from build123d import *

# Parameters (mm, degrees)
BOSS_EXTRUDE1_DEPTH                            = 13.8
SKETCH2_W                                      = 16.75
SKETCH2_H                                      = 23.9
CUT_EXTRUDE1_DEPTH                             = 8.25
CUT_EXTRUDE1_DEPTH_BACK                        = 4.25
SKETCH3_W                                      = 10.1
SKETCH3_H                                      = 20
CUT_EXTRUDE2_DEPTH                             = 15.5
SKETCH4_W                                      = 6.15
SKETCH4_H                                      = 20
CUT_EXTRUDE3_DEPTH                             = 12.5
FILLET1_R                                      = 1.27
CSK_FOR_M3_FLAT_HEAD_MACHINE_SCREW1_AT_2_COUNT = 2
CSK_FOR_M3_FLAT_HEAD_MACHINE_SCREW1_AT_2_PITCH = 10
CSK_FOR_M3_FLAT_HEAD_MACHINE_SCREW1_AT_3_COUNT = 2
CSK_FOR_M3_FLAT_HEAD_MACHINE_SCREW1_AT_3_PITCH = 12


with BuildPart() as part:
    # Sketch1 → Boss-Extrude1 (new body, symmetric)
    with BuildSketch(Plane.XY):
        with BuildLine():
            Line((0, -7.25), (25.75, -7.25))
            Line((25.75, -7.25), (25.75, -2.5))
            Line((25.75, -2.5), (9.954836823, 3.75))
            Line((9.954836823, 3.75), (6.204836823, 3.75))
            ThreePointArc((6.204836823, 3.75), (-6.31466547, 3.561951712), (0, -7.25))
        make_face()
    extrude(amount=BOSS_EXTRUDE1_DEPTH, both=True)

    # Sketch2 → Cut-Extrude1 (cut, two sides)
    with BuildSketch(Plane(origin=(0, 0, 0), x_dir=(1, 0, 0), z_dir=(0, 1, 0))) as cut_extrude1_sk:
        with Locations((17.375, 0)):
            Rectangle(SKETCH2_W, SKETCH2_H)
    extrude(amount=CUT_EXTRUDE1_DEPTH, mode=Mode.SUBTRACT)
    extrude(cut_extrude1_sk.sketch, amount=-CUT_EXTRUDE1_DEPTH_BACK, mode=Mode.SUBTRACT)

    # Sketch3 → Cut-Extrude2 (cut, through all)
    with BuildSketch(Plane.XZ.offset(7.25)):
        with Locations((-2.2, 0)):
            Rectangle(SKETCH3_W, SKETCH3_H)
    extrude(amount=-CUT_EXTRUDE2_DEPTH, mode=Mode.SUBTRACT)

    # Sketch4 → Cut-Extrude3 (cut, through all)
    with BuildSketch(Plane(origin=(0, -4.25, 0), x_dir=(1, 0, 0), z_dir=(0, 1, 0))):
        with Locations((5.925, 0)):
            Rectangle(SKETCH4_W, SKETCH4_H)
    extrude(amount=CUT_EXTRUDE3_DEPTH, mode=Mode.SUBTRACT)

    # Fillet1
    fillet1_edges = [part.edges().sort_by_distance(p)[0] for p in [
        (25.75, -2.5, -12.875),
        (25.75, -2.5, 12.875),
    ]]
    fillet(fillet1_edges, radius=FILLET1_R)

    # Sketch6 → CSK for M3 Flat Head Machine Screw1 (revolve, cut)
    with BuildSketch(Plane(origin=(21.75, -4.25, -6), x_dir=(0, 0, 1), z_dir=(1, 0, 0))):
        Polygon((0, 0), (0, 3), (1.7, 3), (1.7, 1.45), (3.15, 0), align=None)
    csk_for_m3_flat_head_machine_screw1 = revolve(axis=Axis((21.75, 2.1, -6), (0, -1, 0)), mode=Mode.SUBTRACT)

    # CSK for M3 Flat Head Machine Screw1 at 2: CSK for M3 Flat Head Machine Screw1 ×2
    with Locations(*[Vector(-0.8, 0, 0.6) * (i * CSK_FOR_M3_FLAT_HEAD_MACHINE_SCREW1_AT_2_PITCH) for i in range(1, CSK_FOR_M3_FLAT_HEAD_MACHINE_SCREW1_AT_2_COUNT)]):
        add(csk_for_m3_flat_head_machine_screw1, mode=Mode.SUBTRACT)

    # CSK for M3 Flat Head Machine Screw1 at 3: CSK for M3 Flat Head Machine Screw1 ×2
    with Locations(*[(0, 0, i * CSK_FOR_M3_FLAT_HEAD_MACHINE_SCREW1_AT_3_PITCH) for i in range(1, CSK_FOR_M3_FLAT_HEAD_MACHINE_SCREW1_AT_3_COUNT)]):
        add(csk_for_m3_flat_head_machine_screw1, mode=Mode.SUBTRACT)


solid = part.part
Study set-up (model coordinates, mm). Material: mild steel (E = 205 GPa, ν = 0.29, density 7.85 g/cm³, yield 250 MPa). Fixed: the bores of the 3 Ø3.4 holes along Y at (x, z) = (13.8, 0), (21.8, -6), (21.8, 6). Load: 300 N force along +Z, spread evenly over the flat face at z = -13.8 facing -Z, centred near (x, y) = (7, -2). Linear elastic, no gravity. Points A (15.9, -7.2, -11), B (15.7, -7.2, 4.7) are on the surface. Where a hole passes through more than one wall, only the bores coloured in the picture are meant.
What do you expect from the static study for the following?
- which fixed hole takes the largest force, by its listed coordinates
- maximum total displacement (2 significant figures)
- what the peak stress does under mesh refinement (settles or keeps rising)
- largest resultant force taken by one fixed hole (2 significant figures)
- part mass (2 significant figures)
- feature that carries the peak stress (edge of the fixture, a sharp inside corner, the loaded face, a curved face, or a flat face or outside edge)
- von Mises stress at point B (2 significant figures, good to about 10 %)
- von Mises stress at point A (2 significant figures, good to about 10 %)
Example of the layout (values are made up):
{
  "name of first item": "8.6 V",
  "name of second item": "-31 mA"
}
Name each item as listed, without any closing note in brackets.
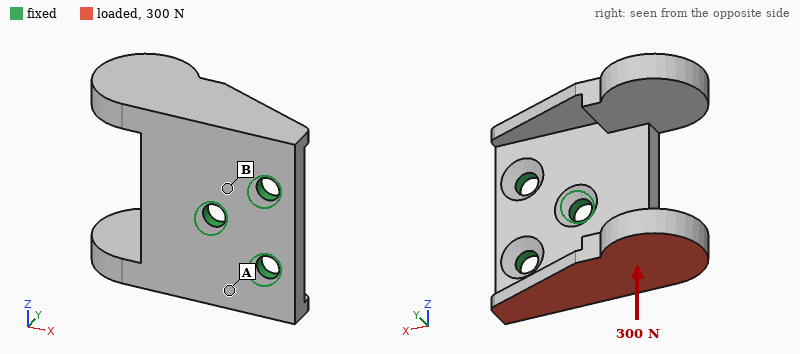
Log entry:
{
  "which fixed hole takes the largest force, by its listed coordinates": "(13.8, 0)",
  "maximum total displacement": "38 µm",
  "what the peak stress does under mesh refinement": "keeps rising",
  "largest resultant force taken by one fixed hole": "290 N",
  "part mass": "27 g",
  "feature that carries the peak stress": "edge of the fixture",
  "von Mises stress at point B": "10 MPa",
  "von Mises stress at point A": "30 MPa"
}
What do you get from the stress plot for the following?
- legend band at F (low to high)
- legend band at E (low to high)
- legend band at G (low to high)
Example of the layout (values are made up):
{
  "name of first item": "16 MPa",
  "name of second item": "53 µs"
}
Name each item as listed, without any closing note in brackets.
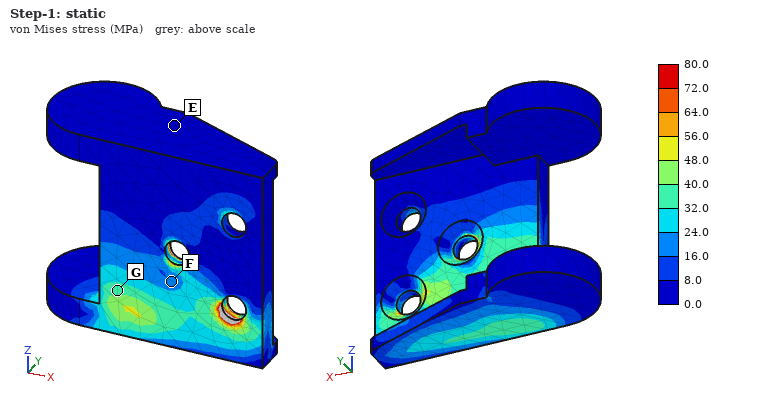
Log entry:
{
  "legend band at F": "16.0 to 24.0 MPa",
  "legend band at E": "0.0 to 8.0 MPa",
  "legend band at G": "32.0 to 40.0 MPa"
}
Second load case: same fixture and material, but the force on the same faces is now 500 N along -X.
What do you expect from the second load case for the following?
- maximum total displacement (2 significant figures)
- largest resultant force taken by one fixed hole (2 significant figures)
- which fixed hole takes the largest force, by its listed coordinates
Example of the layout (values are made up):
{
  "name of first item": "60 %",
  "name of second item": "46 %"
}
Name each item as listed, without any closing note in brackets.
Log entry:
{
  "maximum total displacement": "35 µm",
  "largest resultant force taken by one fixed hole": "550 N",
  "which fixed hole takes the largest force, by its listed coordinates": "(21.8, -6)"
}
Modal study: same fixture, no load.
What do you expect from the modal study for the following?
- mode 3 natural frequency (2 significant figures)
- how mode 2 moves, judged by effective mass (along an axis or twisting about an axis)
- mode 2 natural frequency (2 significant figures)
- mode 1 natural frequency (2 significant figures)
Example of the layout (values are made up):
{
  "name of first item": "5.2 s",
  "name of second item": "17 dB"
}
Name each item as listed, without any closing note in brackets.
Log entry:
{
  "mode 3 natural frequency": "8400 Hz",
  "how mode 2 moves, judged by effective mass": "along Y",
  "mode 2 natural frequency": "4000 Hz",
  "mode 1 natural frequency": "3600 Hz"
}
